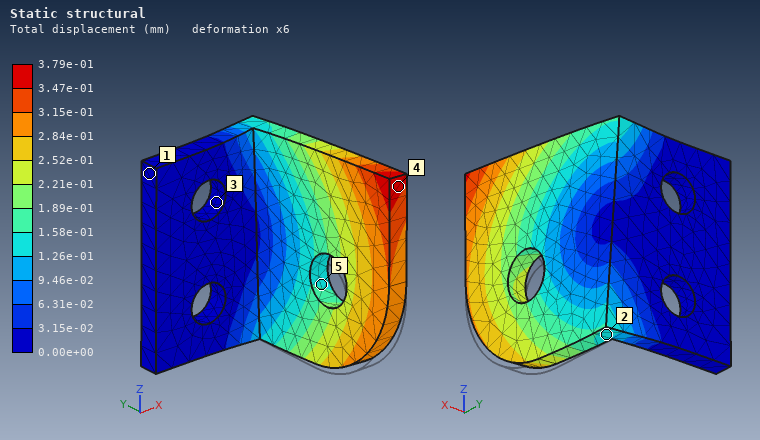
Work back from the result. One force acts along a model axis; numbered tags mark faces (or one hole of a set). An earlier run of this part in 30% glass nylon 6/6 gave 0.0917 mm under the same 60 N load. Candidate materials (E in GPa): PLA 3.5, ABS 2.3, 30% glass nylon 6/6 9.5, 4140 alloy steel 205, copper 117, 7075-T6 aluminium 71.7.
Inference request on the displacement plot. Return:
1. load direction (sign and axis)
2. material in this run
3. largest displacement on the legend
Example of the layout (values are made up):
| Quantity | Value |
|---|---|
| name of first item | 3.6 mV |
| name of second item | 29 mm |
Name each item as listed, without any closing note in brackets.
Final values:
| Quantity | Value |
|---|---|
| load direction | +Z |
| material in this run | ABS |
| largest displacement on the legend | 3.79e-01 mm |
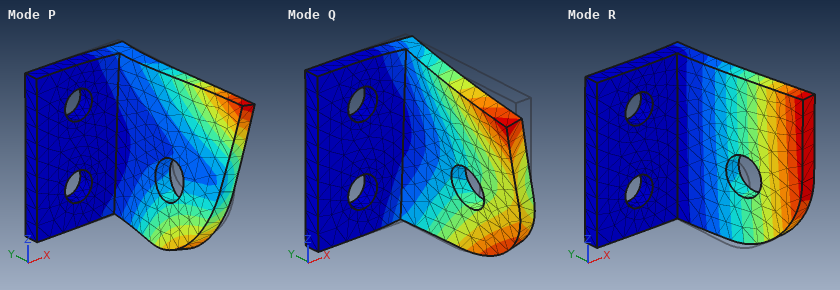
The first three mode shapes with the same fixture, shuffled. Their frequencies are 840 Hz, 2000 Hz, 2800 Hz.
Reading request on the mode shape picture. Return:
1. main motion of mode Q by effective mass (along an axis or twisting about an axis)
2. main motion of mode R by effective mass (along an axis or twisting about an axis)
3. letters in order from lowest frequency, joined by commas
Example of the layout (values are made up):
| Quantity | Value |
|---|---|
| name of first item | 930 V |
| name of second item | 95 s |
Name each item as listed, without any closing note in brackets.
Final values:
| Quantity | Value |
|---|---|
| main motion of mode Q by effective mass | along Z |
| main motion of mode R by effective mass | along X |
| letters in order from lowest frequency, joined by commas | R, Q, P |
